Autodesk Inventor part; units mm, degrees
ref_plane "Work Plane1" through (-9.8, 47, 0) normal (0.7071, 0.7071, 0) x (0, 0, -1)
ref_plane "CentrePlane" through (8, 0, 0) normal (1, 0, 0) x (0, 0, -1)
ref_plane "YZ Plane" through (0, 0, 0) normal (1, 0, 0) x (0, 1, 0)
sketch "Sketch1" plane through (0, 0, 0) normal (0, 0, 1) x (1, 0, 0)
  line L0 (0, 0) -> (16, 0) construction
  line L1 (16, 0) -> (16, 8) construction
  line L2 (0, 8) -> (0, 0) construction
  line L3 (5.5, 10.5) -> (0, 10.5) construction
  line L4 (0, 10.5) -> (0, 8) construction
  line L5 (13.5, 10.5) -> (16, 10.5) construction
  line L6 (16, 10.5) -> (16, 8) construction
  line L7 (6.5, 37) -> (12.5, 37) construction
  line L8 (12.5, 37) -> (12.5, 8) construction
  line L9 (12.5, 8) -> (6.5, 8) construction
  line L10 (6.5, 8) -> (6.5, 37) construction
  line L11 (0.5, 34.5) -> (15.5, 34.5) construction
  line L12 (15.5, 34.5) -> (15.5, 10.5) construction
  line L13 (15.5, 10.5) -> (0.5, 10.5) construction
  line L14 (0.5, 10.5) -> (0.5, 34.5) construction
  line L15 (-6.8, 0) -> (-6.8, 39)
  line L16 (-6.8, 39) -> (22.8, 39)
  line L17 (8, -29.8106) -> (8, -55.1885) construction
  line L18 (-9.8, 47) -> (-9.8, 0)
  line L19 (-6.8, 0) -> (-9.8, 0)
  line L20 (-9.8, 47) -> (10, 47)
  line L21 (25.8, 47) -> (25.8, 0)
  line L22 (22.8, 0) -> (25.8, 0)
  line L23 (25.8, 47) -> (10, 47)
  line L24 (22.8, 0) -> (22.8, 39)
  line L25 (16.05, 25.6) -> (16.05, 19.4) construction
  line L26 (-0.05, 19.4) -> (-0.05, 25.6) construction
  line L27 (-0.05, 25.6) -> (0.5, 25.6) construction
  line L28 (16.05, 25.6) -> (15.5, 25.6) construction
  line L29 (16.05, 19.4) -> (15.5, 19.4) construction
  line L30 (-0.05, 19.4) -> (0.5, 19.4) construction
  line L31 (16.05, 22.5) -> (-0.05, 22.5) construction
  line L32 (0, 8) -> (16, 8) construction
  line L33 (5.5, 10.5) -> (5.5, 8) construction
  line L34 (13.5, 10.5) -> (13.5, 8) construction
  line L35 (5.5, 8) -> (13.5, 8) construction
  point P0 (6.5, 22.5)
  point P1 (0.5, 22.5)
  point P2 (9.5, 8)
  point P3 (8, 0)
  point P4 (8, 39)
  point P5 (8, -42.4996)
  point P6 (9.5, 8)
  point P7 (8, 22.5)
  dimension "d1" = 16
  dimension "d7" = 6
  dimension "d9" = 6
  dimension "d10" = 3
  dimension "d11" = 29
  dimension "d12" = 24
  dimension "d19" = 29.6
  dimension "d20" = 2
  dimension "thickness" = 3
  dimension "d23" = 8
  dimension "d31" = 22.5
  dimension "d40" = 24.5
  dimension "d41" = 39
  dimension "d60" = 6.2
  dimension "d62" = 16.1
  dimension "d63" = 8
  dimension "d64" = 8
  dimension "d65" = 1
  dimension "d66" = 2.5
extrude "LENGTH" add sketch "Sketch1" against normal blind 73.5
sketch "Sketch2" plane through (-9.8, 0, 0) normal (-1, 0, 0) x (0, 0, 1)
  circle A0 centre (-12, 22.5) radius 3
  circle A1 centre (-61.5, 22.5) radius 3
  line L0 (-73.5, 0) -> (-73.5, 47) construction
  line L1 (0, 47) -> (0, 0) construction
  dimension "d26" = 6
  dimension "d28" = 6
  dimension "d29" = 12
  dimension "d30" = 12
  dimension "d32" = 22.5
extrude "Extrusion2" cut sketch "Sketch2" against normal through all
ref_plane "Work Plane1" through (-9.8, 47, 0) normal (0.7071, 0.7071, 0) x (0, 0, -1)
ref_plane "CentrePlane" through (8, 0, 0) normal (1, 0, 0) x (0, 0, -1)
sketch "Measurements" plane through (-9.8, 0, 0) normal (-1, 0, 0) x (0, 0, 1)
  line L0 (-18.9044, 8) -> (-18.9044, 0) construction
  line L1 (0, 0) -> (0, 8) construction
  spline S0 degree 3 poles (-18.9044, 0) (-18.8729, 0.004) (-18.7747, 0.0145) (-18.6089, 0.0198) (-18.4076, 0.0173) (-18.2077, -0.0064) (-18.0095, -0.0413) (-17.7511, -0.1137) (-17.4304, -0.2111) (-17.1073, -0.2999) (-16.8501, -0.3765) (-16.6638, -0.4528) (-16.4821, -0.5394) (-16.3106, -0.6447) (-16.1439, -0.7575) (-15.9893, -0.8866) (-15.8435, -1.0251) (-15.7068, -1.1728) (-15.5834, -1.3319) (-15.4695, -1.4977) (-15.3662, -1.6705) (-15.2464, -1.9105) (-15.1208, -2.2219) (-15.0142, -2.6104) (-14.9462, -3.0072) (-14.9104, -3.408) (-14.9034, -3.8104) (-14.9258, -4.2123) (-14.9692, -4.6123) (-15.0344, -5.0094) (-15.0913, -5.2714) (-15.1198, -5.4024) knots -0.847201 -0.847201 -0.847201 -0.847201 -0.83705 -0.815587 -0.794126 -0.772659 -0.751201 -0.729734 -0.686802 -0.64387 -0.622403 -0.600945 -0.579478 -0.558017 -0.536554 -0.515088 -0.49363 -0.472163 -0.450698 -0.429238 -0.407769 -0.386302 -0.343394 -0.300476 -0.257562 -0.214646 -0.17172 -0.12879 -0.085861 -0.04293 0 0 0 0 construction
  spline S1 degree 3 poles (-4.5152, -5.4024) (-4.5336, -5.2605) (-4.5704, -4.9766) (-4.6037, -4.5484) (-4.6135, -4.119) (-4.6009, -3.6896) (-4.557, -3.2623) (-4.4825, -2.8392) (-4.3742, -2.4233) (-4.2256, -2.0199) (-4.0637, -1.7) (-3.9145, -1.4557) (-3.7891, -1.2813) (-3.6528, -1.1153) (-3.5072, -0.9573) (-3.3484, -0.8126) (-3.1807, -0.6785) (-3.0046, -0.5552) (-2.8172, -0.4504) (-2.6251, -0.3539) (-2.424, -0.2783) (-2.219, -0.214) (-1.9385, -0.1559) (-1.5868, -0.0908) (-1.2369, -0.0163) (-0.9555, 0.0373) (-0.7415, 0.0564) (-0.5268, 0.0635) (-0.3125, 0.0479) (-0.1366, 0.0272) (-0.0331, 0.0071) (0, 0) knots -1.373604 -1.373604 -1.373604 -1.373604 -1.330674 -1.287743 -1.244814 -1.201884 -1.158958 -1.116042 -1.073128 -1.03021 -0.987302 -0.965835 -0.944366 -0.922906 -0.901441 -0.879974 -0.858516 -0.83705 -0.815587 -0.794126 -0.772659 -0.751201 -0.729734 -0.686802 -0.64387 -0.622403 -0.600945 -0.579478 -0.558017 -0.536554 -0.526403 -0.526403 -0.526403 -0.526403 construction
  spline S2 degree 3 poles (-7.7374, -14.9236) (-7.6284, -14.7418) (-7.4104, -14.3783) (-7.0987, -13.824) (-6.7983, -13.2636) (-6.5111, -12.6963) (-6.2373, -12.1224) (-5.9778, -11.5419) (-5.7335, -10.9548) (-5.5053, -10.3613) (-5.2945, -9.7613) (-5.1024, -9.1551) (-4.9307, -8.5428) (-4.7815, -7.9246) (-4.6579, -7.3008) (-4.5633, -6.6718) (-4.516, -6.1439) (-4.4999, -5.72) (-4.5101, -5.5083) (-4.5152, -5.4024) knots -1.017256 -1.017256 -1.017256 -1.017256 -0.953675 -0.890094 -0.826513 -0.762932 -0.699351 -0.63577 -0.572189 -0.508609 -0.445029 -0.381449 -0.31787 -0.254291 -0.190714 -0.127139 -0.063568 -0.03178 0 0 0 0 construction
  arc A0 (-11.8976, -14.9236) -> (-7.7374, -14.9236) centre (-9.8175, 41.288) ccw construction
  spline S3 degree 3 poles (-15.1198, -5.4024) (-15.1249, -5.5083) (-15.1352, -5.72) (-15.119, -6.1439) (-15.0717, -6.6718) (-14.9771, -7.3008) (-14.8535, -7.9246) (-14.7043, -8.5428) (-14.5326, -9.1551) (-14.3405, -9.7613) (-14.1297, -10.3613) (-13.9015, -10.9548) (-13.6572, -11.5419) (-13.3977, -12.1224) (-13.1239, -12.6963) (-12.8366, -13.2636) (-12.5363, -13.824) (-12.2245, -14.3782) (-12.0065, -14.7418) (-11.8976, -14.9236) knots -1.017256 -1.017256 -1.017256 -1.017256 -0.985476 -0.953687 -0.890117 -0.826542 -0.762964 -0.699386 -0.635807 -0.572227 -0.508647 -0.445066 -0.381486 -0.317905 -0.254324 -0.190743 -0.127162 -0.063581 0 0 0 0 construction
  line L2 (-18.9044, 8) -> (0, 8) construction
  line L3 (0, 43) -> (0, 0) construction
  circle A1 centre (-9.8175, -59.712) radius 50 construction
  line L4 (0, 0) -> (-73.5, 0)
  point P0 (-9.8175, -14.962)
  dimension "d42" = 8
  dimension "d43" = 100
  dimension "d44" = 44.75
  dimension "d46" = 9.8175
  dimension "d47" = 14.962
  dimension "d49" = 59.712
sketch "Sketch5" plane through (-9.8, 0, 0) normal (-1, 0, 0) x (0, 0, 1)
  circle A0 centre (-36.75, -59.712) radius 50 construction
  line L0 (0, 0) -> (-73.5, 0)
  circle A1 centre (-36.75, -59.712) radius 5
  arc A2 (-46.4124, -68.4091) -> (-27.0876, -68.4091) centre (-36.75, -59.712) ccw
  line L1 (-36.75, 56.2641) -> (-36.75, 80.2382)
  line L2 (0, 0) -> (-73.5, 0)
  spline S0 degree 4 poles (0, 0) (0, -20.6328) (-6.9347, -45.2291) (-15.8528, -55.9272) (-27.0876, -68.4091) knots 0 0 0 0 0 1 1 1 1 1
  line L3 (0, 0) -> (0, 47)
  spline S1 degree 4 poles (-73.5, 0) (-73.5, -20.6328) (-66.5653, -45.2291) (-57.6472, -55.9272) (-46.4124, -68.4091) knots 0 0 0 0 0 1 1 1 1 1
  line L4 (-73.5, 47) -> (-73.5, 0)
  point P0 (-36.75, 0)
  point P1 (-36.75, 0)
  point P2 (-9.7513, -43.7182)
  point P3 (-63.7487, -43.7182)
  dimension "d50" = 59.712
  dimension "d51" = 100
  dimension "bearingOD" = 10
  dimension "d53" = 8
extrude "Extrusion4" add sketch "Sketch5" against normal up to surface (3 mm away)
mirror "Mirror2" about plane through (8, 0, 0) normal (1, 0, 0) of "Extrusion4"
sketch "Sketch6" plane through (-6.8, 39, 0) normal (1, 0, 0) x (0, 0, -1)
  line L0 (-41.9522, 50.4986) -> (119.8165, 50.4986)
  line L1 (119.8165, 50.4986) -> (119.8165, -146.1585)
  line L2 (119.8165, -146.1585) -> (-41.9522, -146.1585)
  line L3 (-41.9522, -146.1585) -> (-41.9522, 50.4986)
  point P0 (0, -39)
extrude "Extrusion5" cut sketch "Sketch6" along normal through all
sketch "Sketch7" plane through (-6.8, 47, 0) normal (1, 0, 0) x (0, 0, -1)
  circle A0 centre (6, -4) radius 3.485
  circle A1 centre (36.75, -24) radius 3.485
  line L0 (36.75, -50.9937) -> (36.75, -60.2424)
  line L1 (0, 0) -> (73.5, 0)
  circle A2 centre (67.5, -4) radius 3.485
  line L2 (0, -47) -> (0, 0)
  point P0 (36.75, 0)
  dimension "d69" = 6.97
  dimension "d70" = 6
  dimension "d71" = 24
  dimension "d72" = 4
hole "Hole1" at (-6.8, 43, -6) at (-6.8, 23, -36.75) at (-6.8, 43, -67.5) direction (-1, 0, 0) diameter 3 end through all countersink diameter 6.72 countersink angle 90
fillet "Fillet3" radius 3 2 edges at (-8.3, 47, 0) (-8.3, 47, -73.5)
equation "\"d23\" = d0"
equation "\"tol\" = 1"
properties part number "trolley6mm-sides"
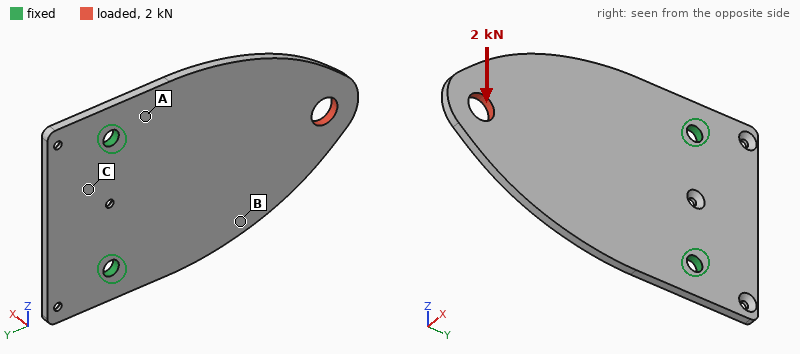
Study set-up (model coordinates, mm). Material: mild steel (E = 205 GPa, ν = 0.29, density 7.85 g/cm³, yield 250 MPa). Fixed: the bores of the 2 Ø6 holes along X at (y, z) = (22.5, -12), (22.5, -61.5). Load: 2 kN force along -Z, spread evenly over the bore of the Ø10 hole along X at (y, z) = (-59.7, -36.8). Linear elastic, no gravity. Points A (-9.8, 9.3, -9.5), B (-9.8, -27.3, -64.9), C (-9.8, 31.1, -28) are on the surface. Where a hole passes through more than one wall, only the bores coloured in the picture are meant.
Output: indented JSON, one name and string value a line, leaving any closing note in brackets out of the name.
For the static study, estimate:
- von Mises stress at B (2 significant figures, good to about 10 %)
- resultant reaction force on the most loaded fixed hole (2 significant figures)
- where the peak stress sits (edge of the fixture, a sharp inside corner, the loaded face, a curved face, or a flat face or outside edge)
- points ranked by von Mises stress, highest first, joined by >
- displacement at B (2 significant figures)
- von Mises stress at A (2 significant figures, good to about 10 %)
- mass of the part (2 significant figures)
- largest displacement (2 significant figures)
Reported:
{
  "von Mises stress at B": "28 MPa",
  "resultant reaction force on the most loaded fixed hole": "3.3 kN",
  "where the peak stress sits": "edge of the fixture",
  "points ranked by von Mises stress, highest first, joined by >": "A > B > C",
  "displacement at B": "19 µm",
  "von Mises stress at A": "44 MPa",
  "mass of the part": "170 g",
  "largest displacement": "41 µm"
}
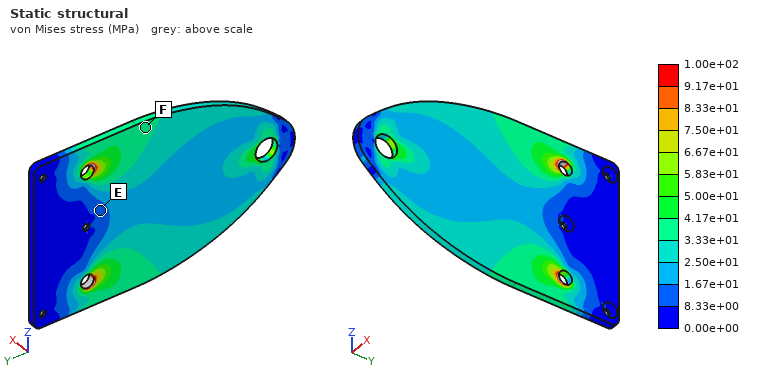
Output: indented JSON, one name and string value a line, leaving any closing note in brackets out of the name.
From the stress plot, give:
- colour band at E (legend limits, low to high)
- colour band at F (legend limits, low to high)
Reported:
{
  "colour band at E": "8.33e+00 to 1.67e+01 MPa",
  "colour band at F": "3.33e+01 to 4.17e+01 MPa"
}
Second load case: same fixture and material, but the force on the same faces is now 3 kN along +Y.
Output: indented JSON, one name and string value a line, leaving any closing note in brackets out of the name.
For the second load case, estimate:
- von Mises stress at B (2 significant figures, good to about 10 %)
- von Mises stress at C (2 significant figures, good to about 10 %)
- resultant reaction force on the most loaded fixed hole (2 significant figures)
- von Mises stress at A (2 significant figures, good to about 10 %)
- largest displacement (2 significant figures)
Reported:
{
  "von Mises stress at B": "13 MPa",
  "von Mises stress at C": "5.9 MPa",
  "resultant reaction force on the most loaded fixed hole": "1.5 kN",
  "von Mises stress at A": "19 MPa",
  "largest displacement": "11 µm"
}
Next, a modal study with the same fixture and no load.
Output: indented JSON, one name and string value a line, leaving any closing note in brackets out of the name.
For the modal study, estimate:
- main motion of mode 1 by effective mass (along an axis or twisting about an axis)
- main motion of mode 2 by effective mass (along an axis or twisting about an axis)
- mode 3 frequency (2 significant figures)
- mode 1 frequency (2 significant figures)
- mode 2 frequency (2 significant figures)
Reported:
{
  "main motion of mode 1 by effective mass": "along X",
  "main motion of mode 2 by effective mass": "twisting about Y",
  "mode 3 frequency": "2000 Hz",
  "mode 1 frequency": "380 Hz",
  "mode 2 frequency": "1400 Hz"
}
